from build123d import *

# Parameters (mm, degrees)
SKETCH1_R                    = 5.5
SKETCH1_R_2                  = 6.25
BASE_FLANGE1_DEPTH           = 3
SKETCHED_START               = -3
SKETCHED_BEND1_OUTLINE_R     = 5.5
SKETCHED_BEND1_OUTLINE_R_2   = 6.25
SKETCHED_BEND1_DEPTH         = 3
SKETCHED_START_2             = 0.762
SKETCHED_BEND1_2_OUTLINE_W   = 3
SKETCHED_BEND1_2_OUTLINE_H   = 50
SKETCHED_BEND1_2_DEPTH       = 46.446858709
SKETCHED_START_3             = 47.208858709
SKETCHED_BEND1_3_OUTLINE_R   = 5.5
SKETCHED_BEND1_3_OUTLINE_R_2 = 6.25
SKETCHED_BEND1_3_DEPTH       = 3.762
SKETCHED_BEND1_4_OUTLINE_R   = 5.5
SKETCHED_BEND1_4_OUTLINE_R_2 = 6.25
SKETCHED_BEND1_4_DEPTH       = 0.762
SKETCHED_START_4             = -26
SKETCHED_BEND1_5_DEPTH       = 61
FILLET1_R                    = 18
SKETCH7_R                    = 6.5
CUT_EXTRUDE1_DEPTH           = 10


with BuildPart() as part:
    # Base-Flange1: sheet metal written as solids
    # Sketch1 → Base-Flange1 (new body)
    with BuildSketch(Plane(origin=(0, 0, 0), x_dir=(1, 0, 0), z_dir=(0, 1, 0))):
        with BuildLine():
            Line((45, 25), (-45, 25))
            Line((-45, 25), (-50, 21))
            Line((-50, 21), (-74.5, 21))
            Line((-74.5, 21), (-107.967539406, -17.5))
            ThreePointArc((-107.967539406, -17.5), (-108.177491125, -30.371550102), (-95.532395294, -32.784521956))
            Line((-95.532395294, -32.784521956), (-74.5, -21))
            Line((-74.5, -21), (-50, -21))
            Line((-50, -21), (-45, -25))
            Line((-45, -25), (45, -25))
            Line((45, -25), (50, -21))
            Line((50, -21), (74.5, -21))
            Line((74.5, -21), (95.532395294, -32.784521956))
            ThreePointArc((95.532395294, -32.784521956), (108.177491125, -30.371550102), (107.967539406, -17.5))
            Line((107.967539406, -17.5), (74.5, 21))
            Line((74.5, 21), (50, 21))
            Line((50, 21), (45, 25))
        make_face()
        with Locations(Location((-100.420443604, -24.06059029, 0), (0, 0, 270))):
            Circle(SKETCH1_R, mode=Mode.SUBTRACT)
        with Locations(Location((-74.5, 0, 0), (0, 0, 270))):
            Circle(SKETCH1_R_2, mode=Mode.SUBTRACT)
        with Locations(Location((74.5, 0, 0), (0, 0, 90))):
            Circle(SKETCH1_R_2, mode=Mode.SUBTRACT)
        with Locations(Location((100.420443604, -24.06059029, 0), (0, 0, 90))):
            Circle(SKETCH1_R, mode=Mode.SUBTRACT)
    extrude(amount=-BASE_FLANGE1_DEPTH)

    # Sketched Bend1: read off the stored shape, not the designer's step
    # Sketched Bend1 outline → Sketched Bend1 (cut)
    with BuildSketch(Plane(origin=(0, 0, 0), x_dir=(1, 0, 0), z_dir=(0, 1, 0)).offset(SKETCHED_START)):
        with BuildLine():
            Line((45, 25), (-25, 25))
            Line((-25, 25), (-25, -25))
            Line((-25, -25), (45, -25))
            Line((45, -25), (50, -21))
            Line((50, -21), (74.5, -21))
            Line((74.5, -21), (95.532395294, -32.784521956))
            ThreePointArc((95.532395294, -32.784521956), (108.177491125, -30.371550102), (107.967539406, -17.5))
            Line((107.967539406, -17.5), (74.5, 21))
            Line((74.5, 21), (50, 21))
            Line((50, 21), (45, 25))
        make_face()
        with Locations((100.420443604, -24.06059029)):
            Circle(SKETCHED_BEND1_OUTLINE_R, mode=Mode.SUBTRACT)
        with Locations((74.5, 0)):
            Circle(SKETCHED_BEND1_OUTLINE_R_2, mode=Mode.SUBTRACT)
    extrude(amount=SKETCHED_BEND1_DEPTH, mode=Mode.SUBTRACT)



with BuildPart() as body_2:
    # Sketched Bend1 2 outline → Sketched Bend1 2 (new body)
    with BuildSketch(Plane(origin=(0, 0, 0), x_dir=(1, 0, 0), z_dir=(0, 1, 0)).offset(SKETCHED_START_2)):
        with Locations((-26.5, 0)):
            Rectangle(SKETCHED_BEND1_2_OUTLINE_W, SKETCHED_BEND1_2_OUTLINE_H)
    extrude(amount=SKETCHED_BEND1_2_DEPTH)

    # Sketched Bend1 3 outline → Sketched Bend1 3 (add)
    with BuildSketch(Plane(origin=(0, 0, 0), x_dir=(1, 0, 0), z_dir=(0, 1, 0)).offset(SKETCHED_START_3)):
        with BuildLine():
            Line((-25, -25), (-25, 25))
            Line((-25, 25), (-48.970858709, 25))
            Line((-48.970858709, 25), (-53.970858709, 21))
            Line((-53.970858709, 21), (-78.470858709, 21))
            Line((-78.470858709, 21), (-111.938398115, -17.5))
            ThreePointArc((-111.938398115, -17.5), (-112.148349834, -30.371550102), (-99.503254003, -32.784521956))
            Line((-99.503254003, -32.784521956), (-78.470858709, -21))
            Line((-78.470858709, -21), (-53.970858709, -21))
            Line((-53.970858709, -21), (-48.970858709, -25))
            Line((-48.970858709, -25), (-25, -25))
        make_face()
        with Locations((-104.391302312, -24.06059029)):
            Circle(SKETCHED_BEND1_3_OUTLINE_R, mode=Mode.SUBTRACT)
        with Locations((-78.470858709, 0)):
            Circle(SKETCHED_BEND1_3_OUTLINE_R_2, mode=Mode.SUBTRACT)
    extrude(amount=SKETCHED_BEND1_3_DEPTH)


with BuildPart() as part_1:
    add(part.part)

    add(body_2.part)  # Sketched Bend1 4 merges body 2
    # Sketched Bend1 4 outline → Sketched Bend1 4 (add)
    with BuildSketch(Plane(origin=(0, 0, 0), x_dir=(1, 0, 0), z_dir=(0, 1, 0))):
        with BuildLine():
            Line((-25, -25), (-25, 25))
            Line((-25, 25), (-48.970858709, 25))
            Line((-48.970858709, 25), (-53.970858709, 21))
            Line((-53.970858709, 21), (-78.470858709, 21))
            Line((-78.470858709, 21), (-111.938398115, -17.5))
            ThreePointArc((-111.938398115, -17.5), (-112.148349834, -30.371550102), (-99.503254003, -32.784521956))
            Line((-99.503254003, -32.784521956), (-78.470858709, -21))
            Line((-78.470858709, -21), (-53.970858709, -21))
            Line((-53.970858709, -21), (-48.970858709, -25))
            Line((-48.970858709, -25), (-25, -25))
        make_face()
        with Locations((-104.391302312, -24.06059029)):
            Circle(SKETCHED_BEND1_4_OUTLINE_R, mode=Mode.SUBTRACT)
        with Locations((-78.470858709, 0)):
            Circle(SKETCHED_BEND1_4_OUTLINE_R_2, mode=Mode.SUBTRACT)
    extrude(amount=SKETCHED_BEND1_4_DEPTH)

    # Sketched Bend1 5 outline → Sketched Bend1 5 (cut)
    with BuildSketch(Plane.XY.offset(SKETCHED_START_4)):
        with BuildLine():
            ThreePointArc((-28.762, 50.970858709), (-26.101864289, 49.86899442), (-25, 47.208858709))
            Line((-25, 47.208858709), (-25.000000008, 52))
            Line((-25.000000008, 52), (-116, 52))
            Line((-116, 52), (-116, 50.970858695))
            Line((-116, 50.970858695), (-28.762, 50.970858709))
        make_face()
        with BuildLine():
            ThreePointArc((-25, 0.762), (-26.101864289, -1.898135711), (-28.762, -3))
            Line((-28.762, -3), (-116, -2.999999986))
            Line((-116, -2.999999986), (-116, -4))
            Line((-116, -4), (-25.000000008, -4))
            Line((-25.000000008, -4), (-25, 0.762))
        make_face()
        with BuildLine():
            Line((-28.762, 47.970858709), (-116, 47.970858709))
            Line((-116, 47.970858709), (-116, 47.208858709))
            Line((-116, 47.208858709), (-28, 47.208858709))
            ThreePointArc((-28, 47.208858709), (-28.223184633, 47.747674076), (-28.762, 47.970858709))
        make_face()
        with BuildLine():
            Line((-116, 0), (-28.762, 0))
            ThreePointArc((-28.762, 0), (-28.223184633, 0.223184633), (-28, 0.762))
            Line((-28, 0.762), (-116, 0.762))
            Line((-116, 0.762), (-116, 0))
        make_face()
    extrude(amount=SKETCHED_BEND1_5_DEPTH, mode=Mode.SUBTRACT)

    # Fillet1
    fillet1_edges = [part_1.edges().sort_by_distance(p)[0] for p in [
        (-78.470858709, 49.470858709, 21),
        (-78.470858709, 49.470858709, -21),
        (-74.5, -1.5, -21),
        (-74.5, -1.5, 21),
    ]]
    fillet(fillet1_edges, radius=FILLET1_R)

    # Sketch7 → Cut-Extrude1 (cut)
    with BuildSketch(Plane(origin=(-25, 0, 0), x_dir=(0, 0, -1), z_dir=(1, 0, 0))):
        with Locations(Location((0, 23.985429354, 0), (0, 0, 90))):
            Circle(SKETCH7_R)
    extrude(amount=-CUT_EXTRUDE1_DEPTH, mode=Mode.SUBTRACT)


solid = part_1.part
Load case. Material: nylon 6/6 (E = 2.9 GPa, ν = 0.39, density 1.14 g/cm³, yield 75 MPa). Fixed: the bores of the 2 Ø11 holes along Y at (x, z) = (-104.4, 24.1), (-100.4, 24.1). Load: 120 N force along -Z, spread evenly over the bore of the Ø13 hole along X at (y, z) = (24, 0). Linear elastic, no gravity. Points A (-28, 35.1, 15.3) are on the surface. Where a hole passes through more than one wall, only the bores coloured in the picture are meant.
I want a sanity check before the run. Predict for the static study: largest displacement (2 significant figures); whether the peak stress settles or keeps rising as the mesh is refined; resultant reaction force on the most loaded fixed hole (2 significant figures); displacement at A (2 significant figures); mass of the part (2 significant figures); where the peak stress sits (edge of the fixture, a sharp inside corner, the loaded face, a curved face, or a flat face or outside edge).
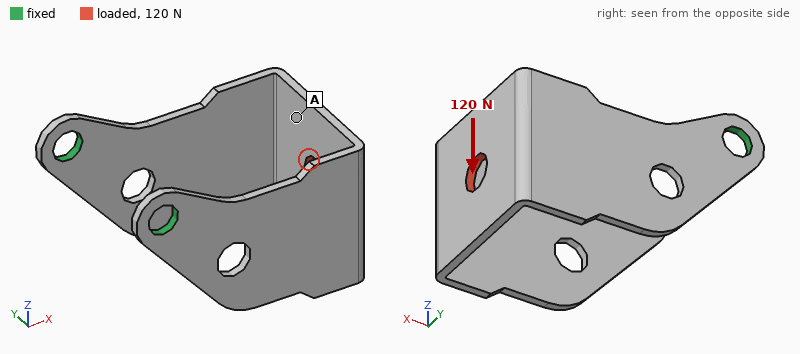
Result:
1.3 mm
keeps rising
60 N
1.0 mm
29 g
edge of the fixture
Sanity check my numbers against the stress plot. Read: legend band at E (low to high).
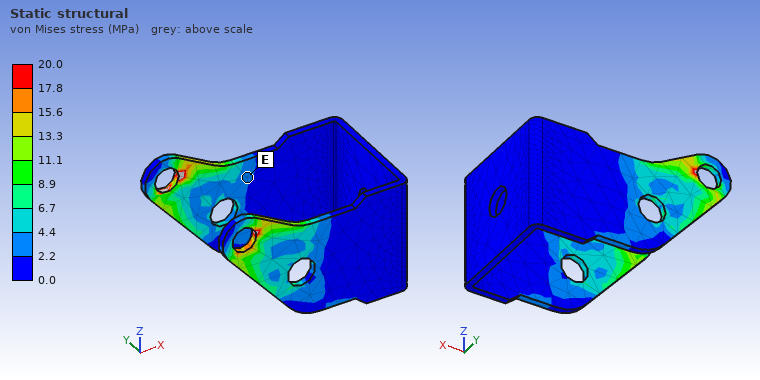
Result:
2.2 to 4.4 MPa
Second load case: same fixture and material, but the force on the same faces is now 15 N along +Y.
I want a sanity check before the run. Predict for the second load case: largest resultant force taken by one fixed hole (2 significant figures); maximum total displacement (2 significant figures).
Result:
15 N
1.4 mm
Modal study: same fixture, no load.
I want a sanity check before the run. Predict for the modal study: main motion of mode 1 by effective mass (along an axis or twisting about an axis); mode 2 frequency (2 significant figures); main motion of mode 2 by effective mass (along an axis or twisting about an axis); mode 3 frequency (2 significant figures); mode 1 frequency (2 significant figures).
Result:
along Y
400 Hz
along Z
440 Hz
130 Hz
